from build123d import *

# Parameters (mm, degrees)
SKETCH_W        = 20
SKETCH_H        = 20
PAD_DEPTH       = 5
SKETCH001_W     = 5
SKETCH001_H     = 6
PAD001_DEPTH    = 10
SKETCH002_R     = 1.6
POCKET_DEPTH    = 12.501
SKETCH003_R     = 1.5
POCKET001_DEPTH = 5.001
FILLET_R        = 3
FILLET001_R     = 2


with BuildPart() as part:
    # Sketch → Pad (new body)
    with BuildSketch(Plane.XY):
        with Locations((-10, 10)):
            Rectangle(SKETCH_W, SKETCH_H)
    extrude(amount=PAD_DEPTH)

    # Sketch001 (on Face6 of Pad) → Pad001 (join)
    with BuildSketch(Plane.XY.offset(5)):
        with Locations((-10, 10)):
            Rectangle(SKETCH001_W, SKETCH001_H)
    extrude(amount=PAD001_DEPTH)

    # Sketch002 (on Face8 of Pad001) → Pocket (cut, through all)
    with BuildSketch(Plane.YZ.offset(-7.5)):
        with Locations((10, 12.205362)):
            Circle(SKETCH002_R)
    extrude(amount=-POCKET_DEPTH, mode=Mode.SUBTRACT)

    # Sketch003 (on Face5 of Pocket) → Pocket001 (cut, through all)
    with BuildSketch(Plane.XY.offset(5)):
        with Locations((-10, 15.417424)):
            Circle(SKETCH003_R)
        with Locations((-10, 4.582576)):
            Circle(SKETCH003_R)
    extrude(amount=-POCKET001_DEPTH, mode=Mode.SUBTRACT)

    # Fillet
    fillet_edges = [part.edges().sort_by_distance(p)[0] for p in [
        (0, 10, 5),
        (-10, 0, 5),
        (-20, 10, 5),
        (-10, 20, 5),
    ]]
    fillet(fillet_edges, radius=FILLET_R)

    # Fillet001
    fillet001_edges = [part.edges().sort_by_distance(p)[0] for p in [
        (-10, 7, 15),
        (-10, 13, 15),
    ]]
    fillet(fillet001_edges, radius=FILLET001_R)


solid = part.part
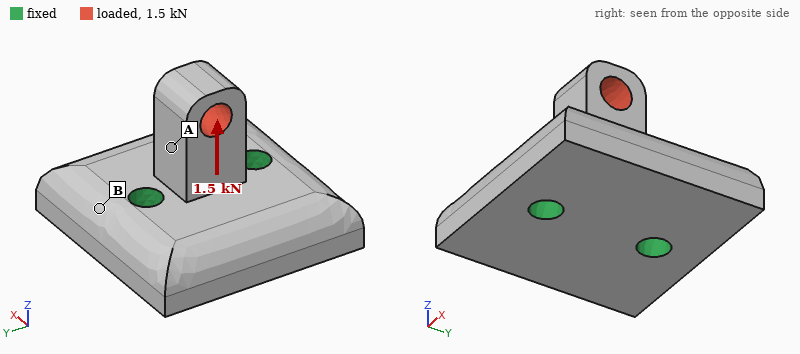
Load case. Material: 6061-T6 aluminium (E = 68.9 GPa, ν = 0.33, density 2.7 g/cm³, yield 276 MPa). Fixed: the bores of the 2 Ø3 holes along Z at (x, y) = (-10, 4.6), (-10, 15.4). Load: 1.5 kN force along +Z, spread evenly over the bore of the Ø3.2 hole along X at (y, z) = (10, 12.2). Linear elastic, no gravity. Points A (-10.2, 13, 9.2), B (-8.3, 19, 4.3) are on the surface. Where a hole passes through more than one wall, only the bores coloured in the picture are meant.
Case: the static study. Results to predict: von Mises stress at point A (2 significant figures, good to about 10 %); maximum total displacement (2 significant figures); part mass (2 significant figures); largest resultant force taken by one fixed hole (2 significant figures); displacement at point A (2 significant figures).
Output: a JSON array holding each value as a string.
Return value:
["69 MPa", "14 µm", "5.5 g", "770 N", "6.5 µm"]
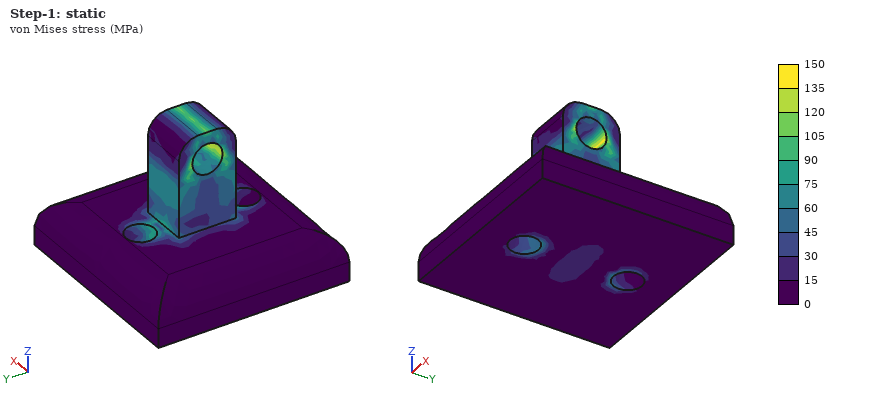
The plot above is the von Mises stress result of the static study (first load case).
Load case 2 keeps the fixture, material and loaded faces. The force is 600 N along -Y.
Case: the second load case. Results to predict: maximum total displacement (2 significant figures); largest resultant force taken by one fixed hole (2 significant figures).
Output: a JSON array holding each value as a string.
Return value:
["43 µm", "660 N"]
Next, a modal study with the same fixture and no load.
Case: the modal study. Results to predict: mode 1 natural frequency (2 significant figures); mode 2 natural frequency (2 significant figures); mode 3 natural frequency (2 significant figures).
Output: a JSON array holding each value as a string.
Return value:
["28 kHz", "37 kHz", "41 kHz"]
